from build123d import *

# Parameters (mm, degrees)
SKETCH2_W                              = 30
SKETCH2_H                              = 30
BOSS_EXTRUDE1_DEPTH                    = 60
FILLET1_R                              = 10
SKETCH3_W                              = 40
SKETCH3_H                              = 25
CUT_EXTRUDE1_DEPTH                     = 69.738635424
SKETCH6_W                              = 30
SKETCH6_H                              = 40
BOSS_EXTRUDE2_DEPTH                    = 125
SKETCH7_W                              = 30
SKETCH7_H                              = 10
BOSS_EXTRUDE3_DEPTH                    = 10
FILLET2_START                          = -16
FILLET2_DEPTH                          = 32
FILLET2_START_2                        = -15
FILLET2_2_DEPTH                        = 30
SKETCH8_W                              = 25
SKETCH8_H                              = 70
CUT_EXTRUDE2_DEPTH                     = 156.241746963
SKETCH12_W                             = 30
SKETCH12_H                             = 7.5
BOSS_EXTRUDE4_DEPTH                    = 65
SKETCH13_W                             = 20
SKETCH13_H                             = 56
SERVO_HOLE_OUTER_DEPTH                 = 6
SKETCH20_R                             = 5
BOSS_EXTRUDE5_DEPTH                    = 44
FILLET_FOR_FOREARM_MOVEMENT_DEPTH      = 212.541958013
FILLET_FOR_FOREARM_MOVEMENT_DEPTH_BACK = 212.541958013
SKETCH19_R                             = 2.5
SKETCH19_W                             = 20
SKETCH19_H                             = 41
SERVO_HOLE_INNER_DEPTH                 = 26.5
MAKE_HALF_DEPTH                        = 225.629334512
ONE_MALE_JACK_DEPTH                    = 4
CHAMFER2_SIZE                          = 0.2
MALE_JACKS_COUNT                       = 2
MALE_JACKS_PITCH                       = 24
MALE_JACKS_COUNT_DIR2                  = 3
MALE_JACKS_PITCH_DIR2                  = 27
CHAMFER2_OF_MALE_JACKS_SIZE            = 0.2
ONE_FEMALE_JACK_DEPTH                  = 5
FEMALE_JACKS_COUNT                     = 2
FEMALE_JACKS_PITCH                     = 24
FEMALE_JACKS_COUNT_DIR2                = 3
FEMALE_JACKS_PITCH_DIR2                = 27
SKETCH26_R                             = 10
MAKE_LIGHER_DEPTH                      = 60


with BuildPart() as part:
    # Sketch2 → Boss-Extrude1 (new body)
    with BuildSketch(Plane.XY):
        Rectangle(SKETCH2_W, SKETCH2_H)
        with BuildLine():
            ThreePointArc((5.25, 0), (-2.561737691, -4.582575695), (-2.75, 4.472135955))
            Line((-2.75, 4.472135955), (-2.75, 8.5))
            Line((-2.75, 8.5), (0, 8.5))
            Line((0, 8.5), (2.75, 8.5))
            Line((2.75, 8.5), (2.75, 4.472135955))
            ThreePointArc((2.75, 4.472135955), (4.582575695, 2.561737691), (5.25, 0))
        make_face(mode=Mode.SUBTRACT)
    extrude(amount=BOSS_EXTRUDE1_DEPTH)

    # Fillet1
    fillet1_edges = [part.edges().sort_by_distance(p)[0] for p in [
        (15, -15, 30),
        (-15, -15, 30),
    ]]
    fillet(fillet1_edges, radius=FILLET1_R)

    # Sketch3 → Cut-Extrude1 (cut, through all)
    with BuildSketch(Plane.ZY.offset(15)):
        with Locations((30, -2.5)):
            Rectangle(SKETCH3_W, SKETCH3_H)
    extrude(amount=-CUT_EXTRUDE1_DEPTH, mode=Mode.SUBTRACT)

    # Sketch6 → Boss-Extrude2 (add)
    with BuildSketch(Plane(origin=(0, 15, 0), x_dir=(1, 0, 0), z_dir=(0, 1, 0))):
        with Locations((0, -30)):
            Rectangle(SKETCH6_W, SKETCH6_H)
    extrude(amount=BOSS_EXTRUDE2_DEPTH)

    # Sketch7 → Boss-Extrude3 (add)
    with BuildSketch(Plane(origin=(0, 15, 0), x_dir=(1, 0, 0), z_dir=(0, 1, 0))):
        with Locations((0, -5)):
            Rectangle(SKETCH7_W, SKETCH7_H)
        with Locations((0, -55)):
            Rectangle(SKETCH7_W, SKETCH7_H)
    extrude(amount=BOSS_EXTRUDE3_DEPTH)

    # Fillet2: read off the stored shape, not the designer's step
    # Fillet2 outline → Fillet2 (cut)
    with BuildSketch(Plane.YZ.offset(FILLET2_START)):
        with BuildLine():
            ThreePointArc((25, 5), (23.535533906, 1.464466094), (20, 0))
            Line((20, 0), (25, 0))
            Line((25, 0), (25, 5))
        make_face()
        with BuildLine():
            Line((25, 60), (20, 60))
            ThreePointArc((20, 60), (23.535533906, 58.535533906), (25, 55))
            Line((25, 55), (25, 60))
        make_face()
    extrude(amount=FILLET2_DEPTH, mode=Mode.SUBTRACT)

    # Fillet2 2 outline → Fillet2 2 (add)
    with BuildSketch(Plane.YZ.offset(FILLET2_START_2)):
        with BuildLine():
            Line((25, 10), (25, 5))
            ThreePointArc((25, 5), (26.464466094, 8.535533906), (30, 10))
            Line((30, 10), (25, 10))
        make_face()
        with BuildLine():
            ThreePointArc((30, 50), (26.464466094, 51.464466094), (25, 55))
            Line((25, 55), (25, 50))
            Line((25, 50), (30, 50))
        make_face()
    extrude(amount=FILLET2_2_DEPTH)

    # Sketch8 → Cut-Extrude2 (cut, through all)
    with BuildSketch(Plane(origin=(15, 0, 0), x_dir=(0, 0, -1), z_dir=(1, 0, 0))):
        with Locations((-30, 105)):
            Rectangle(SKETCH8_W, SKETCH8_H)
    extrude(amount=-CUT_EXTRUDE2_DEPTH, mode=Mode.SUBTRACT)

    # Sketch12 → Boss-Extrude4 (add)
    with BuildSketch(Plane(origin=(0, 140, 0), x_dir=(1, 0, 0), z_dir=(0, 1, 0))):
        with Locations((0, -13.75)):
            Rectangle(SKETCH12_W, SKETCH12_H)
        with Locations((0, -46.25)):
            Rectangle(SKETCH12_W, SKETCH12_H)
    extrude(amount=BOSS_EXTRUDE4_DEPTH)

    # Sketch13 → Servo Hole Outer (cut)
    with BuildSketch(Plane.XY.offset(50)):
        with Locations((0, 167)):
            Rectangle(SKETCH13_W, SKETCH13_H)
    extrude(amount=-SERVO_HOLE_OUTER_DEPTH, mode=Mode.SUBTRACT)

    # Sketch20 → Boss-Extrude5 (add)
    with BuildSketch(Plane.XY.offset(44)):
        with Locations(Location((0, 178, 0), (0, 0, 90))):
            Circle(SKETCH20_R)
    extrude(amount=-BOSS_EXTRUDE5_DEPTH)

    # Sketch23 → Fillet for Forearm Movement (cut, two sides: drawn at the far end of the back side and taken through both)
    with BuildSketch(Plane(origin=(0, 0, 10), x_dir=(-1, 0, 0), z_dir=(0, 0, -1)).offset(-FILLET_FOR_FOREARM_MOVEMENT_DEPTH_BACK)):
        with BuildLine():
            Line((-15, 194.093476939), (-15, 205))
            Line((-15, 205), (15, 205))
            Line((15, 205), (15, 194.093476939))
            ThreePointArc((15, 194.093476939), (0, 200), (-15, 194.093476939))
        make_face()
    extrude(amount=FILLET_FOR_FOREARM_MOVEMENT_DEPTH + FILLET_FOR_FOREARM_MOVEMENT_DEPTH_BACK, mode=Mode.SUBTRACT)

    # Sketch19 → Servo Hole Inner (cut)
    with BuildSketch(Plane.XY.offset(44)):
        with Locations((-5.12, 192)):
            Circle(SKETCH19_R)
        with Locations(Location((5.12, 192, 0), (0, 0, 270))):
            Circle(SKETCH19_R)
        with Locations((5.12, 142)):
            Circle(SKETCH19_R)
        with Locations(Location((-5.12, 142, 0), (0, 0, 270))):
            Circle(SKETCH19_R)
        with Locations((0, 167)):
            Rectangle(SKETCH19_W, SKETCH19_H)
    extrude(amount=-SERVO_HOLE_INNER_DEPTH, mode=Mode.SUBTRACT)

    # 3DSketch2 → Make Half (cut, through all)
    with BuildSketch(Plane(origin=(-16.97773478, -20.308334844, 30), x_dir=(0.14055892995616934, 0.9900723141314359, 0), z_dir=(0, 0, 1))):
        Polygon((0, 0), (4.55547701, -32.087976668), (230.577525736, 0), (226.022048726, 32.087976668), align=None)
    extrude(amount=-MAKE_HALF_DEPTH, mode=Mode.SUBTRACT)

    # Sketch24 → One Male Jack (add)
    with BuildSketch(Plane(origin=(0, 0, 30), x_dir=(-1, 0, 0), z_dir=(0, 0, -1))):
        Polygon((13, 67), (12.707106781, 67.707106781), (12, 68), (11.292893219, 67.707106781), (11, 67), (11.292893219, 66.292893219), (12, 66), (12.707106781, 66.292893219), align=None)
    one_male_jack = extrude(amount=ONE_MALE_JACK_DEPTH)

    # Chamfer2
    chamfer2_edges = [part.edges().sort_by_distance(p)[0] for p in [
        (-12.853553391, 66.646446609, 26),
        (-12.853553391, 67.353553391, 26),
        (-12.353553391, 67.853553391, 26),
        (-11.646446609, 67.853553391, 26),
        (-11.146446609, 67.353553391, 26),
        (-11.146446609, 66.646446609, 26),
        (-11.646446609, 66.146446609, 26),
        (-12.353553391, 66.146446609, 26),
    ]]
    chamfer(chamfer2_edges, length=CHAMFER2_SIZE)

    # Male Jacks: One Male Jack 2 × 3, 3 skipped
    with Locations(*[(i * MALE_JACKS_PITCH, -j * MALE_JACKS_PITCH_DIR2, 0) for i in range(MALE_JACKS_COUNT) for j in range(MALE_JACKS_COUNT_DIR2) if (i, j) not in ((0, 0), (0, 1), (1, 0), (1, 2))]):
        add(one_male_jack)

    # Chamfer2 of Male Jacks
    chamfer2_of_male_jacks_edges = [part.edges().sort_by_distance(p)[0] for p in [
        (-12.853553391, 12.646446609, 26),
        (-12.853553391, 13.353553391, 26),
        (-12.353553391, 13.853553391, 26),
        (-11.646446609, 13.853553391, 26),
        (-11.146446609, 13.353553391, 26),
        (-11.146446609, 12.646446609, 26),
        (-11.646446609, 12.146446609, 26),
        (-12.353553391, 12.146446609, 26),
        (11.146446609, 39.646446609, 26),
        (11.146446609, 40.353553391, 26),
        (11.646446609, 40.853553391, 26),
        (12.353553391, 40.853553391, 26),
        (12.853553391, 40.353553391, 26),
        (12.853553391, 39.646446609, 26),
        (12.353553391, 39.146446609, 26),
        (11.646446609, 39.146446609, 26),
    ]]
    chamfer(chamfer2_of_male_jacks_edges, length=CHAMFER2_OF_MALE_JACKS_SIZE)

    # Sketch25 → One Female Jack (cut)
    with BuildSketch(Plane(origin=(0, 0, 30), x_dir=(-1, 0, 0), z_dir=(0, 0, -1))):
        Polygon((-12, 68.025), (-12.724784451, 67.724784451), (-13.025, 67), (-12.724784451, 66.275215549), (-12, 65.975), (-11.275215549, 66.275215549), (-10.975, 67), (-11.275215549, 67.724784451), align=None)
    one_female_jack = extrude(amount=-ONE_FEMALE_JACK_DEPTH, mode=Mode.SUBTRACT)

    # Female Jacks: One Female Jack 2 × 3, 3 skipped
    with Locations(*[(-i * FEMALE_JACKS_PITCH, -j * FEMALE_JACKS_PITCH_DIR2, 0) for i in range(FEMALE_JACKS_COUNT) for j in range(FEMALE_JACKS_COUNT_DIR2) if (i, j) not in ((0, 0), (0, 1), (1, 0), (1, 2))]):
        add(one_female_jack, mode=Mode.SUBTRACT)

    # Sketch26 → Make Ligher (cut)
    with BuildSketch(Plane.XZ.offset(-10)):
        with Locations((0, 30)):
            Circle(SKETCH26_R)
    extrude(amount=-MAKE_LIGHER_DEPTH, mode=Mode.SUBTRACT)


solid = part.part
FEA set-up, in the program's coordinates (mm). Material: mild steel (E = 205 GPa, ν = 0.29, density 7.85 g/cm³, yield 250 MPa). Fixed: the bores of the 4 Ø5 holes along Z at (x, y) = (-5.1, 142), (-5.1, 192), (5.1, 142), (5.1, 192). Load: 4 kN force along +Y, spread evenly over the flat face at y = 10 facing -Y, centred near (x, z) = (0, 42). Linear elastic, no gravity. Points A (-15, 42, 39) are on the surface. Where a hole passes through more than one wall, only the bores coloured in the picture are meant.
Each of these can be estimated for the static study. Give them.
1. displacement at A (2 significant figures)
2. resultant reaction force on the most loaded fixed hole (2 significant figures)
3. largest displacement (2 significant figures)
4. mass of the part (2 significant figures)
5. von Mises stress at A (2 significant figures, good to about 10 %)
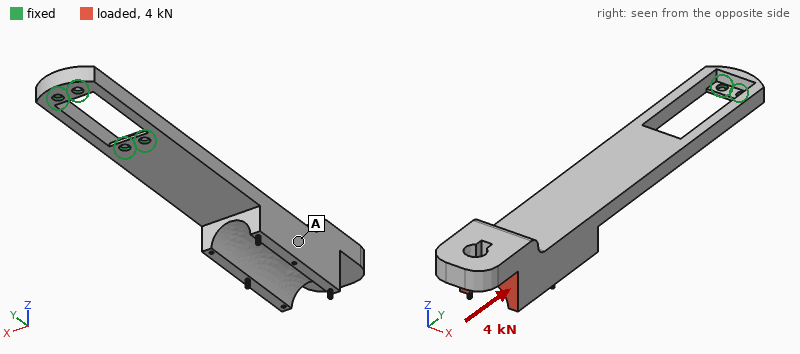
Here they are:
0.43 mm
2.0 kN
0.79 mm
450 g
9.2 MPa
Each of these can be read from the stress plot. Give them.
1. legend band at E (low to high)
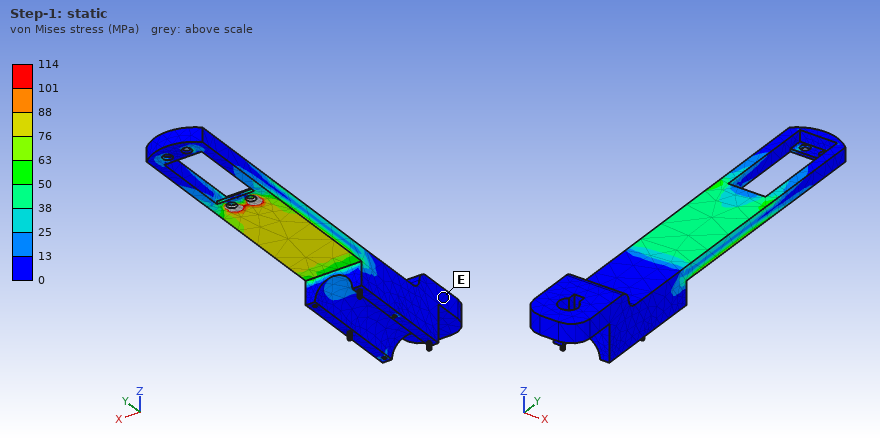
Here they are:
0 to 13 MPa
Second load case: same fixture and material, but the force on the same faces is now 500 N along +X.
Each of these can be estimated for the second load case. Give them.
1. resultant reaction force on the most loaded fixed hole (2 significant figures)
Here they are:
3.0 kN
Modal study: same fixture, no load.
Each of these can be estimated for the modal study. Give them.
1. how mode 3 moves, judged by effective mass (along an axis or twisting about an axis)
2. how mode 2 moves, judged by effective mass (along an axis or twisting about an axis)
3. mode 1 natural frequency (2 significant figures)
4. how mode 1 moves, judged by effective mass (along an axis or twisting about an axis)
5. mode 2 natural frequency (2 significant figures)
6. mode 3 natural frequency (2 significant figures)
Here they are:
twisting about Y
along X
150 Hz
along Z
530 Hz
1300 Hz
